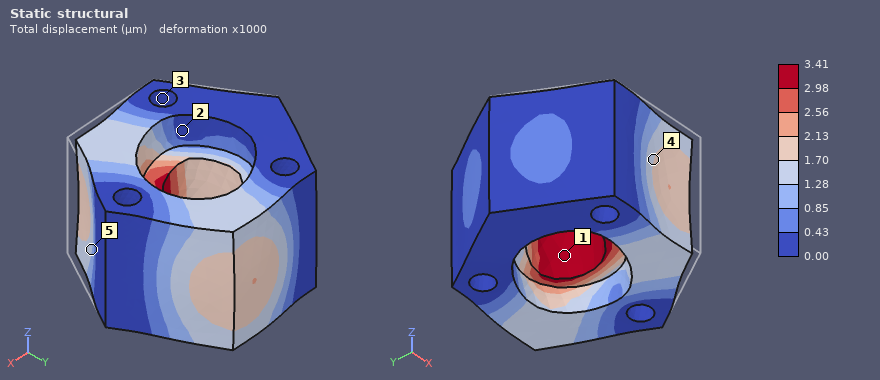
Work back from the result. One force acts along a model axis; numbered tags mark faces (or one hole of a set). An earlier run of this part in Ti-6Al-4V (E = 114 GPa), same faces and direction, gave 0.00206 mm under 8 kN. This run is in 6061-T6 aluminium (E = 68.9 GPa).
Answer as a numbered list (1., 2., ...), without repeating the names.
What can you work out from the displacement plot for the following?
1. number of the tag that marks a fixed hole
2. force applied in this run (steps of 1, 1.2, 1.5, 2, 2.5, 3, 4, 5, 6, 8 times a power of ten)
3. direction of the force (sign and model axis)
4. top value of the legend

1. 3
2. 8 kN
3. +Y
4. 3.41 µm
